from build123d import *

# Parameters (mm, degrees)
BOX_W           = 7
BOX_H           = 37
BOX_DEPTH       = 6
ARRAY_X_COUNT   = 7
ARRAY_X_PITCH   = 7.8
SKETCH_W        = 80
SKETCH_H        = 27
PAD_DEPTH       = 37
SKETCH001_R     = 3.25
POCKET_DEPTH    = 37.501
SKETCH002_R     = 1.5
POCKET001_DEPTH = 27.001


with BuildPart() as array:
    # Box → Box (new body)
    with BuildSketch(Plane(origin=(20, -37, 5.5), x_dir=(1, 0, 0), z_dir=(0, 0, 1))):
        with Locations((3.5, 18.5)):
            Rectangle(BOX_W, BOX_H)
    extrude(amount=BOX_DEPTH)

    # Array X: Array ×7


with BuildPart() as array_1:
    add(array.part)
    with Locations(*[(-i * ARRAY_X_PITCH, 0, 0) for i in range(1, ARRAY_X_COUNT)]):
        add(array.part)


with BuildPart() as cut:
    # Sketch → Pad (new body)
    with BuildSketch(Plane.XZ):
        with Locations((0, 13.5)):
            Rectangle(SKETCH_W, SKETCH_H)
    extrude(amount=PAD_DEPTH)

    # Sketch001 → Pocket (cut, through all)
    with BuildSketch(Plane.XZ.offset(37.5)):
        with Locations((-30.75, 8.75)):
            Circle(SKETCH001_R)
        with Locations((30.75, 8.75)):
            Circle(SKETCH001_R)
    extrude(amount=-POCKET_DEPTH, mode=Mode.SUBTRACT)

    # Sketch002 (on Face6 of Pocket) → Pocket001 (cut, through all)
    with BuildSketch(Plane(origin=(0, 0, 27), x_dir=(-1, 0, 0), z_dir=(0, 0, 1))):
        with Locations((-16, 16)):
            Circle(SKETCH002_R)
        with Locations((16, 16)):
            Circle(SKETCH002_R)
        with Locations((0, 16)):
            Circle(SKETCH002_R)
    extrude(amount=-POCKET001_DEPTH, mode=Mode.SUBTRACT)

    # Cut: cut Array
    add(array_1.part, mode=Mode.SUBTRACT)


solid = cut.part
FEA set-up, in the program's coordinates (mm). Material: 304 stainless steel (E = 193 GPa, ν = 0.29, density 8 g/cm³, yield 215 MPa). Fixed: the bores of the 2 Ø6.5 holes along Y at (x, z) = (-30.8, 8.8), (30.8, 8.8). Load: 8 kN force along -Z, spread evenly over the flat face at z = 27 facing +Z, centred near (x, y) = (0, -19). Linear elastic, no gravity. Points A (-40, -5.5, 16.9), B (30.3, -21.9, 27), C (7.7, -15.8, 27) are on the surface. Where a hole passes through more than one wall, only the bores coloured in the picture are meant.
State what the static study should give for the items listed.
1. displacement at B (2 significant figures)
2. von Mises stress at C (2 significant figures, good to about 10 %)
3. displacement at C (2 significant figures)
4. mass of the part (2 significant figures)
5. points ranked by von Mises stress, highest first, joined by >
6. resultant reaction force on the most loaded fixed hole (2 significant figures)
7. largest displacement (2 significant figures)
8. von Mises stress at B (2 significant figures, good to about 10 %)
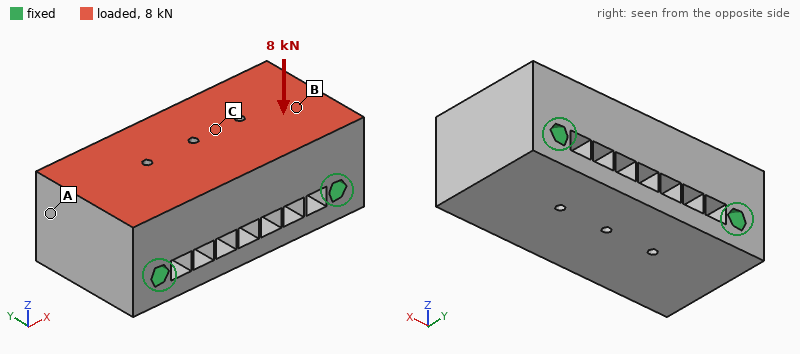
1.0 µm
9.6 MPa
2.9 µm
530 g
C > B > A
4.3 kN
3.4 µm
5.6 MPa
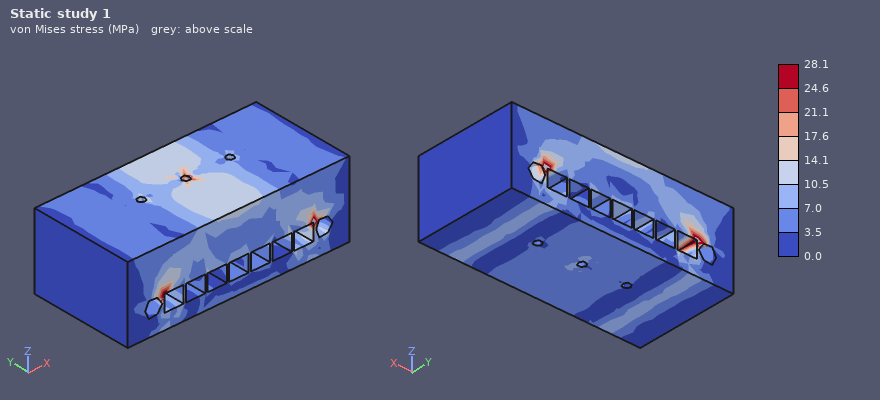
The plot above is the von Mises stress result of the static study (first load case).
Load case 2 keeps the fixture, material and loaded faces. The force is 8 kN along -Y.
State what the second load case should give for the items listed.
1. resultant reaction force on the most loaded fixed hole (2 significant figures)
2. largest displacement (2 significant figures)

4.0 kN
4.6 µm
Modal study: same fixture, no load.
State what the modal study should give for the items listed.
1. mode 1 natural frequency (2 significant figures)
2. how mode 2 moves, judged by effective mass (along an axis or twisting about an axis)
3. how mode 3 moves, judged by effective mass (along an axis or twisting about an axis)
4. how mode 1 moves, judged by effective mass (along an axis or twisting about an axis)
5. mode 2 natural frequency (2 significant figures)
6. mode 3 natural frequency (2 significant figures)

12 kHz
along Y
along Y
along Z
17 kHz
18 kHz
